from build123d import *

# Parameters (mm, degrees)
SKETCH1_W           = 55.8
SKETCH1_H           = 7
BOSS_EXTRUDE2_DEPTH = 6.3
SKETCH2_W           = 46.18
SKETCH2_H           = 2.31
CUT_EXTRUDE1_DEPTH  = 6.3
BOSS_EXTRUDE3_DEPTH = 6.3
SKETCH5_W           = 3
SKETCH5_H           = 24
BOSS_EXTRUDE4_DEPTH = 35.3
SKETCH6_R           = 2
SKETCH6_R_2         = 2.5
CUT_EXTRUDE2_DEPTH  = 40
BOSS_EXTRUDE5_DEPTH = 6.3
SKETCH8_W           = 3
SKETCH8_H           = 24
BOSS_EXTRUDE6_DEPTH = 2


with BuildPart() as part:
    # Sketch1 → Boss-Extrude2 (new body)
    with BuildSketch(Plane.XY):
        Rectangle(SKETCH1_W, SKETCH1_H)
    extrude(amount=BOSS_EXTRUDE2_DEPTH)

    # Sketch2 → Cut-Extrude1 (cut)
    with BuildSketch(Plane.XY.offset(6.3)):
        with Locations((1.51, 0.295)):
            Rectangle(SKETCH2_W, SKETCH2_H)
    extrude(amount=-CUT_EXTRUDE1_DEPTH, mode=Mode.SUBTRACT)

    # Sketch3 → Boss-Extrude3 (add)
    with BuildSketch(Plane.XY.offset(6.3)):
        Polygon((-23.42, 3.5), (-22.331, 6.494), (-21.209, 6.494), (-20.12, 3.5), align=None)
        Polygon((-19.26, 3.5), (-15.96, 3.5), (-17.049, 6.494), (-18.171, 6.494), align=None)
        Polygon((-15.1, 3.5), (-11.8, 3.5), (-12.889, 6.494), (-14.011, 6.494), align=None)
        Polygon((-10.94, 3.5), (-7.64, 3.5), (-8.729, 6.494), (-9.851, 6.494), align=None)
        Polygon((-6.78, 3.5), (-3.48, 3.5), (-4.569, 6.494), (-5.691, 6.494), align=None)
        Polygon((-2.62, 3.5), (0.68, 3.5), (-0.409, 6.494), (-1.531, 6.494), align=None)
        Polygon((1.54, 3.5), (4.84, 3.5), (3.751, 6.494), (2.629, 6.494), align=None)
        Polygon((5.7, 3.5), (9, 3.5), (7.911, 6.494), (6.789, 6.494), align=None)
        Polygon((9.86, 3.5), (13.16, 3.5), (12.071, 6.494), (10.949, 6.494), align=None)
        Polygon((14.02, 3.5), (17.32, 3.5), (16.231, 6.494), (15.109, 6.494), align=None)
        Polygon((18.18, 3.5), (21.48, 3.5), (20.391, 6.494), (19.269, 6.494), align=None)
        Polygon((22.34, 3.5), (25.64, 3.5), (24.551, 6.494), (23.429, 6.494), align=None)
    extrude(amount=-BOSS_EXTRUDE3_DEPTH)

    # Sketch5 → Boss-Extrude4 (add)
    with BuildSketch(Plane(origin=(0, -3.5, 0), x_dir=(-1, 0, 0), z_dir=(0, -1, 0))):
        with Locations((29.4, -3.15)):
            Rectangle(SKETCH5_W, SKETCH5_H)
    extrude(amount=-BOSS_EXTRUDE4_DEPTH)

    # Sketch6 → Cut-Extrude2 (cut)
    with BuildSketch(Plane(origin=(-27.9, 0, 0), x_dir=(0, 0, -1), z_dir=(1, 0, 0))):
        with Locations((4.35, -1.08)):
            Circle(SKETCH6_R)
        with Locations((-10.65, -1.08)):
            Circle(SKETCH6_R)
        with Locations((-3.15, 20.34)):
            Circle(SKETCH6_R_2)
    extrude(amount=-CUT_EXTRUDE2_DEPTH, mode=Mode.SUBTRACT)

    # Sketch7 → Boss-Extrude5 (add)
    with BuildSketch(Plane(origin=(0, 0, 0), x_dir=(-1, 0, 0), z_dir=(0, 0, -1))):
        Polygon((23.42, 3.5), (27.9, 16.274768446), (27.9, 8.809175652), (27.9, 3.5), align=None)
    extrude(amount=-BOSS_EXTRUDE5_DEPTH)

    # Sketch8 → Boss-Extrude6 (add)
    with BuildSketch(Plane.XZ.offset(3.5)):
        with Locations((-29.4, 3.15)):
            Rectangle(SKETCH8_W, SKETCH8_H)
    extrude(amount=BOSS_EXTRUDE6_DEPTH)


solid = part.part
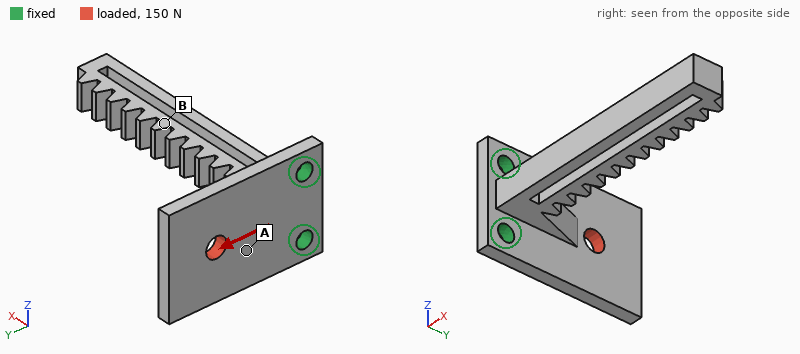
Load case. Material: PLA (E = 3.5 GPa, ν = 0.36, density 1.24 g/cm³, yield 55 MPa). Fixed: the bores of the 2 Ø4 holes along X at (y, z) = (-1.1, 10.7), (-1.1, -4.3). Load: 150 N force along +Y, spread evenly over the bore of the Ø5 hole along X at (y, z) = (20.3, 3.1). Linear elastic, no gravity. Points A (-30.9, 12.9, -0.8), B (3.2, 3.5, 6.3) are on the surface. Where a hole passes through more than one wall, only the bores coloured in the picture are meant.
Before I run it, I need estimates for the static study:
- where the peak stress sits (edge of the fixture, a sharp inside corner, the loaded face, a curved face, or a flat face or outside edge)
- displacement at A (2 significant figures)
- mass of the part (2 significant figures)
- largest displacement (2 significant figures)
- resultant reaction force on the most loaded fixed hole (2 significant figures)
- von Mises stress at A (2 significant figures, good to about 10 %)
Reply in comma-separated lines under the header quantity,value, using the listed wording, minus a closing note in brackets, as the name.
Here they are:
quantity,value
where the peak stress sits,the loaded face
displacement at A,12 µm
mass of the part,6.2 g
largest displacement,35 µm
resultant reaction force on the most loaded fixed hole,76 N
von Mises stress at A,3.0 MPa
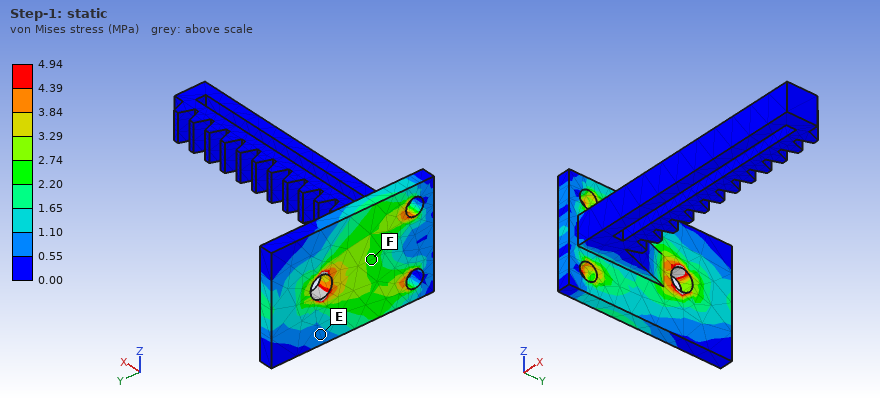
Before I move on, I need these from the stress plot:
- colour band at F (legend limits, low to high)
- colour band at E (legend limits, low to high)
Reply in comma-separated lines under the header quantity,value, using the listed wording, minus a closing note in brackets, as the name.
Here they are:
quantity,value
colour band at F,2.20 to 2.74 MPa
colour band at E,0.55 to 1.10 MPa
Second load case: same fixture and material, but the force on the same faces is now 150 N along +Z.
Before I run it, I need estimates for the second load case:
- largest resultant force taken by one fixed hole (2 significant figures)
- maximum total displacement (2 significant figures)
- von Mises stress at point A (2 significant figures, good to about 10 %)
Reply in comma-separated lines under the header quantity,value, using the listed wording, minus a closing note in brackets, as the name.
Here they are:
quantity,value
largest resultant force taken by one fixed hole,200 N
maximum total displacement,0.12 mm
von Mises stress at point A,5.3 MPa
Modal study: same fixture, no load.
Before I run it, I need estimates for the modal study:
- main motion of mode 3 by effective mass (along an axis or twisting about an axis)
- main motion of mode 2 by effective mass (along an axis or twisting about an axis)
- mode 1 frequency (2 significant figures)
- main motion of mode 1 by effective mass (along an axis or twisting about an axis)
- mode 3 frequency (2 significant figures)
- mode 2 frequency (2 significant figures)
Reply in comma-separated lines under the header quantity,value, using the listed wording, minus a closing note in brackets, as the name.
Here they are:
quantity,value
main motion of mode 3 by effective mass,along X
main motion of mode 2 by effective mass,along Z
mode 1 frequency,330 Hz
main motion of mode 1 by effective mass,along Y
mode 3 frequency,1100 Hz
mode 2 frequency,480 Hz
